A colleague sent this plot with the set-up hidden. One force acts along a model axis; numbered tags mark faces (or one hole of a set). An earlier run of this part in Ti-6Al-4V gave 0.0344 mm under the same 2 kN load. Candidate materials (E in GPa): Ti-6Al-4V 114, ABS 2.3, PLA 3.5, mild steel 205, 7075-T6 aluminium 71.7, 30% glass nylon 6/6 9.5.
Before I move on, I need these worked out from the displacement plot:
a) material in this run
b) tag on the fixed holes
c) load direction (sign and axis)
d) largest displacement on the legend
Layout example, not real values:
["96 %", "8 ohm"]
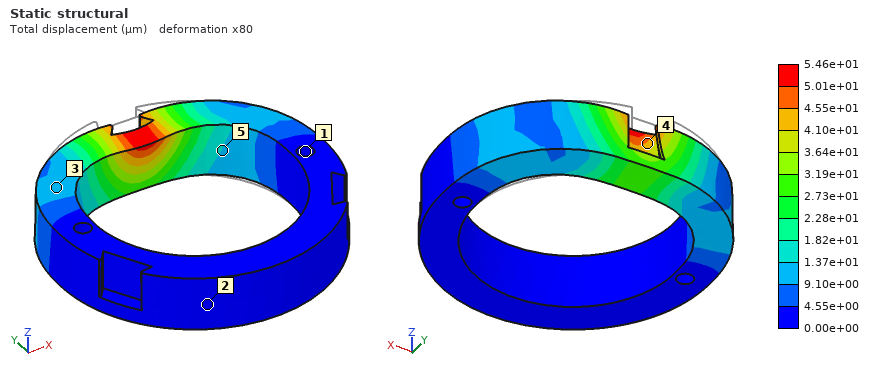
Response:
["7075-T6 aluminium", "1", "-Y", "5.46e+01 µm"]
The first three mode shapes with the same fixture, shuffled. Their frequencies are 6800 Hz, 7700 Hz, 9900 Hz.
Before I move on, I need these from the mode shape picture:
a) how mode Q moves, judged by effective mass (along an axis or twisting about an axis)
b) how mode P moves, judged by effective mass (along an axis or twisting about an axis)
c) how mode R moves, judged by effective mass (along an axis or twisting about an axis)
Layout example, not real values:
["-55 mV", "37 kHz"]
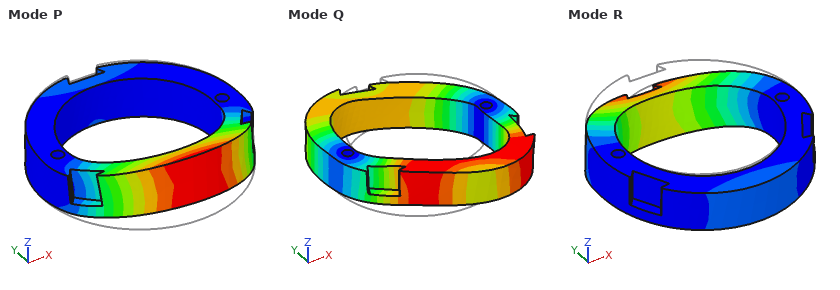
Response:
["twisting about Z", "along Z", "along Z"]
